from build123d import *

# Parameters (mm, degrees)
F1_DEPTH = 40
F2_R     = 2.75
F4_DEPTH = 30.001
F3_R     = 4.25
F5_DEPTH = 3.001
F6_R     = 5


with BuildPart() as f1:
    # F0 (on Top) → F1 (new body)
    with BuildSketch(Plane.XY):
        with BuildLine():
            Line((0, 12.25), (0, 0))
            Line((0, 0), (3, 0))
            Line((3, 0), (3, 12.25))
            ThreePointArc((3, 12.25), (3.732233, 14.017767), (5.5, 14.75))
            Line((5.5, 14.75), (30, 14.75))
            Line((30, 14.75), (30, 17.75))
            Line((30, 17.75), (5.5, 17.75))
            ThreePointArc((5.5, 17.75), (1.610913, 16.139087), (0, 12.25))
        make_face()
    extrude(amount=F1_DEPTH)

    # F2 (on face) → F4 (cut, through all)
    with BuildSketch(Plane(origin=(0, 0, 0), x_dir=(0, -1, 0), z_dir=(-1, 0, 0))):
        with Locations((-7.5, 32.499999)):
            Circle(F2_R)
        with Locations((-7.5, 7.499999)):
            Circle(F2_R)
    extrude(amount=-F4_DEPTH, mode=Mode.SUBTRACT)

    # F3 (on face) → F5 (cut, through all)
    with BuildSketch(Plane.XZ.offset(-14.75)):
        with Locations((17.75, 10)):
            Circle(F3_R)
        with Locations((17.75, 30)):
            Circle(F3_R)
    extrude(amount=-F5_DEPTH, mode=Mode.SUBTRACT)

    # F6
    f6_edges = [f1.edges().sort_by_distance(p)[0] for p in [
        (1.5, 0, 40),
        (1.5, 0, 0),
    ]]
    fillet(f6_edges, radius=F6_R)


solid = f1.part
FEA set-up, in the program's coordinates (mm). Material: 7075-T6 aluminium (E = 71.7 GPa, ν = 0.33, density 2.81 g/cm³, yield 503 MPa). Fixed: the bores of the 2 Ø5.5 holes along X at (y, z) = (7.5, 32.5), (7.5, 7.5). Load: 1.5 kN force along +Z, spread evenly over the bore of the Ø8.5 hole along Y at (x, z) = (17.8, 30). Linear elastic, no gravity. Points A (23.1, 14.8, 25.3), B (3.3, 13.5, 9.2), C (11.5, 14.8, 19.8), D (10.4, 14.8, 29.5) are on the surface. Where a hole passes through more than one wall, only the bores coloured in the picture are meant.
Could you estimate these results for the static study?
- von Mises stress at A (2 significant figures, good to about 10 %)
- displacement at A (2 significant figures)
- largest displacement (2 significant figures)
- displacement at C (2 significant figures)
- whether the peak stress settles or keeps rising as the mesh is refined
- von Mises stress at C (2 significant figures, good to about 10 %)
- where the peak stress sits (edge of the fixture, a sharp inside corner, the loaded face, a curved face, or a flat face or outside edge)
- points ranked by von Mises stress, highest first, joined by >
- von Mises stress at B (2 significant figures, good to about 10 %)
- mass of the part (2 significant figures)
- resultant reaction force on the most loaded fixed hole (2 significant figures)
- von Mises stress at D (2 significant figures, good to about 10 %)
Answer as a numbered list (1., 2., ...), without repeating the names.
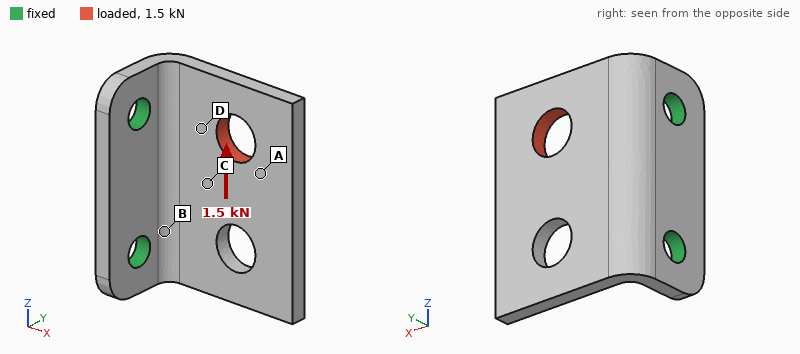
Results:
1. 22 MPa
2. 0.078 mm
3. 0.13 mm
4. 0.034 mm
5. keeps rising
6. 52 MPa
7. edge of the fixture
8. B > D > C > A
9. 100 MPa
10. 13 g
11. 1.2 kN
12. 76 MPa
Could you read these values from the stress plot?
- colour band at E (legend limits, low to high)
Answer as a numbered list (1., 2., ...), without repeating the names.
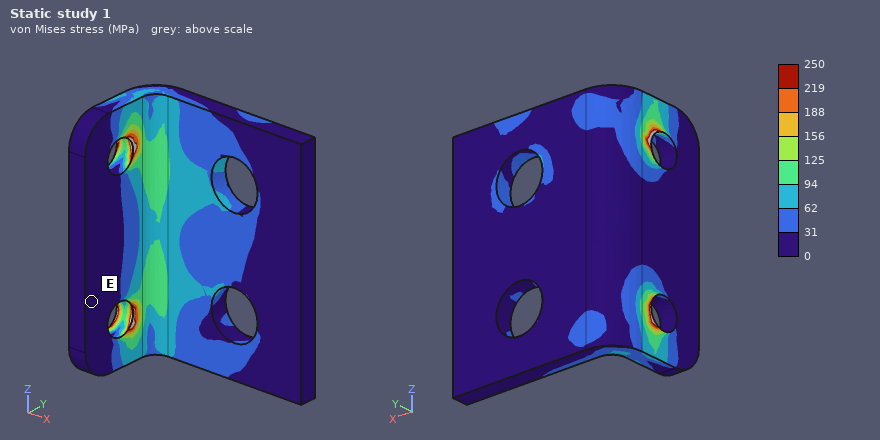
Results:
1. 0 to 31 MPa
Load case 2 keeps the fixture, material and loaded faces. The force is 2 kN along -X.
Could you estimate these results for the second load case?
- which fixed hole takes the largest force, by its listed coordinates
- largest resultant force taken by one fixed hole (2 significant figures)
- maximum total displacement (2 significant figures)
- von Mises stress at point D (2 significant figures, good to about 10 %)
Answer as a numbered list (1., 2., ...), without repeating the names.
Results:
1. (7.5, 32.5)
2. 1.7 kN
3. 0.36 mm
4. 61 MPa
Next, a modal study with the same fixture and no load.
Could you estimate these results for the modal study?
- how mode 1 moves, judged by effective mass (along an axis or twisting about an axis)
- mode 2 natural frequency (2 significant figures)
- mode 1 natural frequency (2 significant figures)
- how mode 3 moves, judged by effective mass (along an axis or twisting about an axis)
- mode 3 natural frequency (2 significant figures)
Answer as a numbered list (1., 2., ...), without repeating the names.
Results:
1. along Y
2. 4700 Hz
3. 2300 Hz
4. along Z
5. 8800 Hz
